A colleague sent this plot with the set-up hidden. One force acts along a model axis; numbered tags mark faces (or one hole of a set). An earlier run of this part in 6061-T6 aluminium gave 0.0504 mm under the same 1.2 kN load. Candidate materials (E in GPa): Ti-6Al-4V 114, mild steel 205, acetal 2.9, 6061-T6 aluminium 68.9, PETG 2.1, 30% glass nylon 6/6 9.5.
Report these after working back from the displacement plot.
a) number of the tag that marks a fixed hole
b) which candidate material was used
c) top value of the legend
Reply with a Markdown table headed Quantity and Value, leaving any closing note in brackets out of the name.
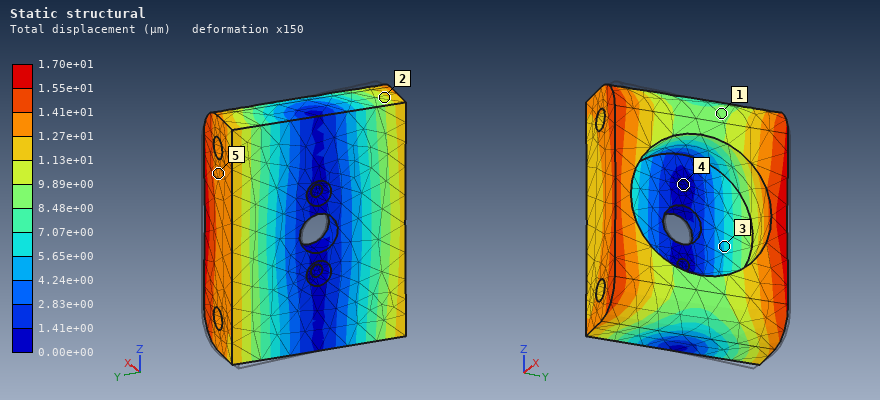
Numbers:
| Quantity | Value |
|---|---|
| number of the tag that marks a fixed hole | 4 |
| which candidate material was used | mild steel |
| top value of the legend | 1.70e+01 µm |
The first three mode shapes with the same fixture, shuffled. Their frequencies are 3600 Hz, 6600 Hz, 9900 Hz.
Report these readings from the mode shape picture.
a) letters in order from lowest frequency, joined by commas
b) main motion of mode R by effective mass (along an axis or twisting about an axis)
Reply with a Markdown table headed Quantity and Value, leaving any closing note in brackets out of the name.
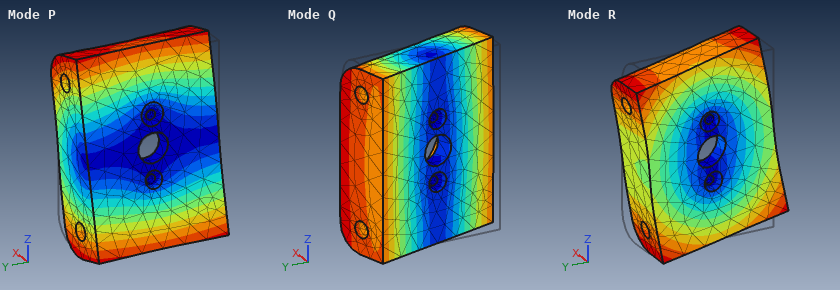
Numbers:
| Quantity | Value |
|---|---|
| letters in order from lowest frequency, joined by commas | Q, P, R |
| main motion of mode R by effective mass | twisting about X |
